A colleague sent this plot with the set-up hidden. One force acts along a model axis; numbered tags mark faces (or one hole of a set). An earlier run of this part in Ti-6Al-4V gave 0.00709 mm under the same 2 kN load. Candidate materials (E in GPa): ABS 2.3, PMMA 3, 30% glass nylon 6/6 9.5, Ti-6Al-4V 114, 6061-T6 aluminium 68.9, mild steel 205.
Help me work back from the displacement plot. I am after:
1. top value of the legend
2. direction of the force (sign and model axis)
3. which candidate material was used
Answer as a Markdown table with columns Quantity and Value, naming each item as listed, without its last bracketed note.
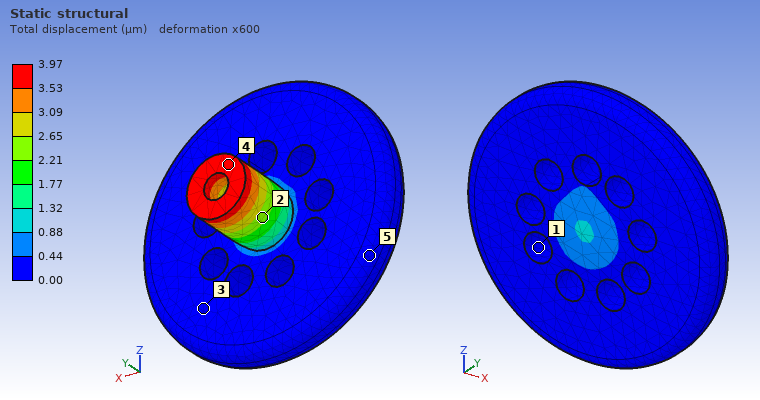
| Quantity | Value |
|---|---|
| top value of the legend | 3.97 µm |
| direction of the force | -Y |
| which candidate material was used | mild steel |
